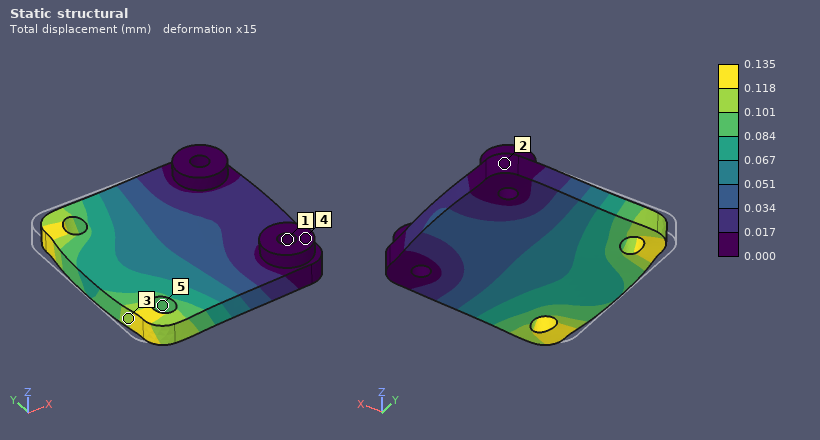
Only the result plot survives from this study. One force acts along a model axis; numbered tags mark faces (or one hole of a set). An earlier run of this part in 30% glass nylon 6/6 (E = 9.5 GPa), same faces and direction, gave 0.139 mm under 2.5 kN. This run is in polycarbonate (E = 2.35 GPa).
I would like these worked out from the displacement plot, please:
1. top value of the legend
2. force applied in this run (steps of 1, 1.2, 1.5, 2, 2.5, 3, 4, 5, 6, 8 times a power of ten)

0.135 mm
600 N
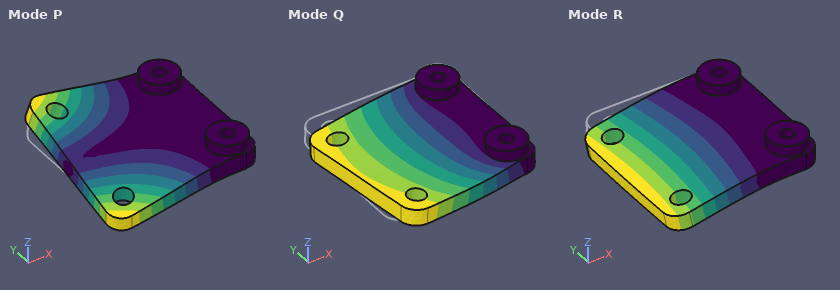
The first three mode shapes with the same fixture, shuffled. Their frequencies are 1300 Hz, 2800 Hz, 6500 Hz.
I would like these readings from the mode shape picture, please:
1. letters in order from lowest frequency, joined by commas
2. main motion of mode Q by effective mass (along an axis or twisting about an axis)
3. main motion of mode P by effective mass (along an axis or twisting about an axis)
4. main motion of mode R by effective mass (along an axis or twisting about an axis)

R, P, Q
along Y
twisting about X
along Z
